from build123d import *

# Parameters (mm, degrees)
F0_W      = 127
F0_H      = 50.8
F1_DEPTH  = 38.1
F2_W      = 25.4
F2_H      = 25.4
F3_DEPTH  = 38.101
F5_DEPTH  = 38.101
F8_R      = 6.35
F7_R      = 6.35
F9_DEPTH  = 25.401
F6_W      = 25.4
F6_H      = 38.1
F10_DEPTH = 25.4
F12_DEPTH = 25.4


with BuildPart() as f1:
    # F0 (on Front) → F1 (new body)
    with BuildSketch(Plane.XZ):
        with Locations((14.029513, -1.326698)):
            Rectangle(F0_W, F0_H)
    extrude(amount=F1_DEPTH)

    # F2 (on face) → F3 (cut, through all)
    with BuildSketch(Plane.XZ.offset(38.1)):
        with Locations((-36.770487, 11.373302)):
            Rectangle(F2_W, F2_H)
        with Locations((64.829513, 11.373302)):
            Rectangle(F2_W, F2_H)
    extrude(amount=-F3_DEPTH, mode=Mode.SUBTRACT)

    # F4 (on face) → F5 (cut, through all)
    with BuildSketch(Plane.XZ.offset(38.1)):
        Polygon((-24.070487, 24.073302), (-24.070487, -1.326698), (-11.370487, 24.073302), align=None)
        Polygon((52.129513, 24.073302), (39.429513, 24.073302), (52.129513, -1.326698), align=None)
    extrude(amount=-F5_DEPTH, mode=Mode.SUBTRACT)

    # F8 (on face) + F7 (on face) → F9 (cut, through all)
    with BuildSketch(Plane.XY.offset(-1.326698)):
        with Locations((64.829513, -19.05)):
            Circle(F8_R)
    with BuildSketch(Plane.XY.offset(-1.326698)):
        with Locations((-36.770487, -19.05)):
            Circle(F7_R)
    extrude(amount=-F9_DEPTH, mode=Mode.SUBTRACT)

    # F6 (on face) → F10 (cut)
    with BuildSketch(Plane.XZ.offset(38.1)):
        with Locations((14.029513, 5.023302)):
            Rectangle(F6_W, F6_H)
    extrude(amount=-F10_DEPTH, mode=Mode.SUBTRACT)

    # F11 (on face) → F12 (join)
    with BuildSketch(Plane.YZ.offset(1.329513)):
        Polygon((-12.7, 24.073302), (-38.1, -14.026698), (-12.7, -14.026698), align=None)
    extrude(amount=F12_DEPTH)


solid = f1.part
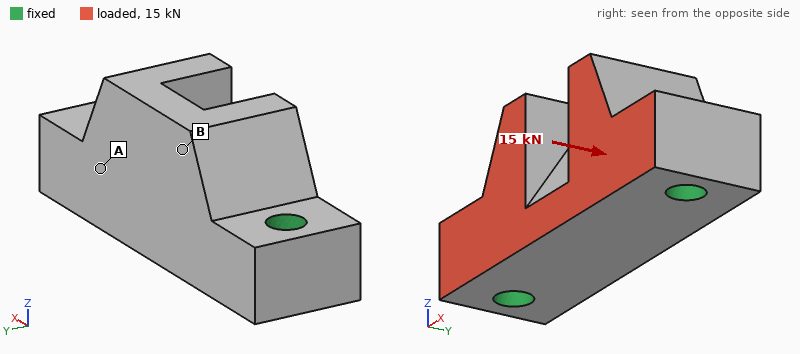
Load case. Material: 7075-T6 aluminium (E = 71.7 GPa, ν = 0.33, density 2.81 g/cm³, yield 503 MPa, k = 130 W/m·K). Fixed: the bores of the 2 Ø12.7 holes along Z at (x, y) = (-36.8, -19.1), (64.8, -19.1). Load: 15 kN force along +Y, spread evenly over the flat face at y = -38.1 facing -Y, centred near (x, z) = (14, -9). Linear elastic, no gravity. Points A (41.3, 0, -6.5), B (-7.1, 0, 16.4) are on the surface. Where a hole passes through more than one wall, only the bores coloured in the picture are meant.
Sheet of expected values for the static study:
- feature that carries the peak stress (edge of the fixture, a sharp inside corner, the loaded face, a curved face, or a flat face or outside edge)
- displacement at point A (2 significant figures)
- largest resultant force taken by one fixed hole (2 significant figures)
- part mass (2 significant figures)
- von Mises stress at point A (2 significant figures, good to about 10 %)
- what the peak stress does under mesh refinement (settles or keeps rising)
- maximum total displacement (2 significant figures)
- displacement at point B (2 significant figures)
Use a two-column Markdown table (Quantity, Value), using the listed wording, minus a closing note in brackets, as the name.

| Quantity | Value |
|---|---|
| feature that carries the peak stress | edge of the fixture |
| displacement at point A | 11 µm |
| largest resultant force taken by one fixed hole | 7.5 kN |
| part mass | 470 g |
| von Mises stress at point A | 8.8 MPa |
| what the peak stress does under mesh refinement | keeps rising |
| maximum total displacement | 23 µm |
| displacement at point B | 18 µm |
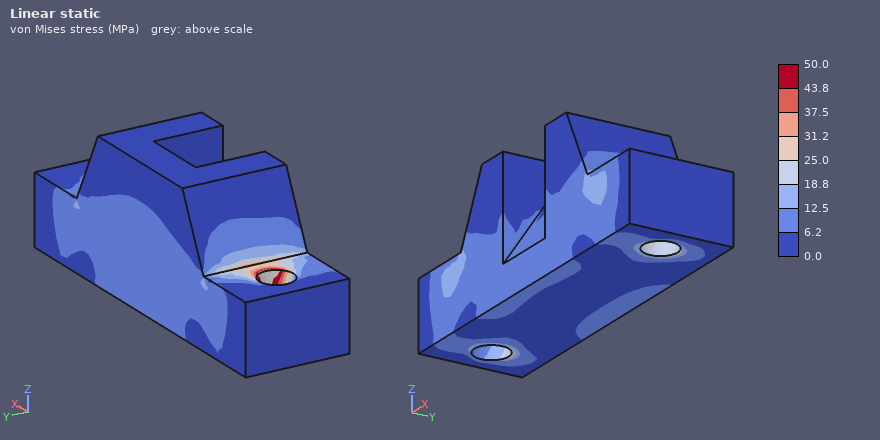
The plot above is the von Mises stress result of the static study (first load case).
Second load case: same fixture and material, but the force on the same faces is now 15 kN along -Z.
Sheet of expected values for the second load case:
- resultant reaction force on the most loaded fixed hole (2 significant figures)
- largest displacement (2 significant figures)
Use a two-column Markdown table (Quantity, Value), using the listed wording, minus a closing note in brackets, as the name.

| Quantity | Value |
|---|---|
| resultant reaction force on the most loaded fixed hole | 7.6 kN |
| largest displacement | 35 µm |
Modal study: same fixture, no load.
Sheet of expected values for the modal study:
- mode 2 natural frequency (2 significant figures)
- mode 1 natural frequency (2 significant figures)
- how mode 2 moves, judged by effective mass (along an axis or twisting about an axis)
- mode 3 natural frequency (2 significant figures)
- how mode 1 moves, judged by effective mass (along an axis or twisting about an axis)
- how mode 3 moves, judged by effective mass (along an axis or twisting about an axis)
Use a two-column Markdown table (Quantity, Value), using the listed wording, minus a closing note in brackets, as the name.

| Quantity | Value |
|---|---|
| mode 2 natural frequency | 9600 Hz |
| mode 1 natural frequency | 6500 Hz |
| how mode 2 moves, judged by effective mass | along Z |
| mode 3 natural frequency | 11 kHz |
| how mode 1 moves, judged by effective mass | along Y |
| how mode 3 moves, judged by effective mass | along Y |
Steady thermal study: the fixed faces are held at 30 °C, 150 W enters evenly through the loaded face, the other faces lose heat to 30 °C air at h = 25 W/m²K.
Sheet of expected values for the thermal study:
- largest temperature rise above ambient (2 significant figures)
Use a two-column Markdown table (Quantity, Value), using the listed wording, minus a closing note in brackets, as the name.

| Quantity | Value |
|---|---|
| largest temperature rise above ambient | 15 K |
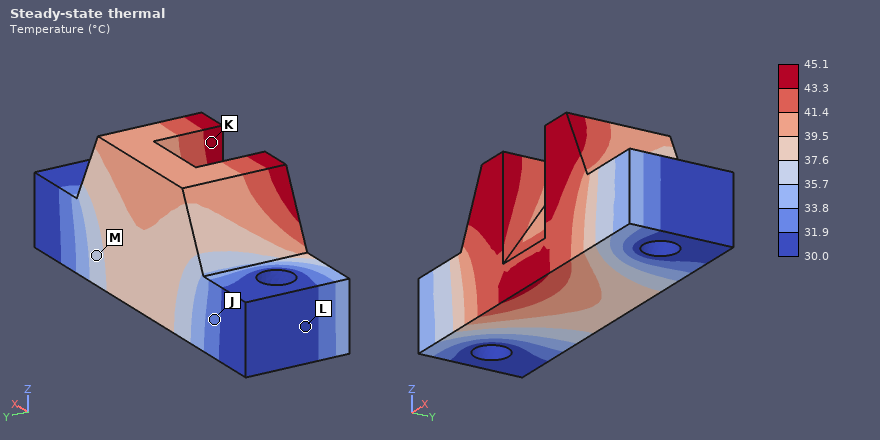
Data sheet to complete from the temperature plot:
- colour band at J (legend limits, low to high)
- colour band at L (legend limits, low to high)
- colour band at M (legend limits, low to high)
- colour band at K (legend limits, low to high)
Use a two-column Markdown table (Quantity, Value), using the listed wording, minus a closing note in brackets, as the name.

| Quantity | Value |
|---|---|
| colour band at J | 31.9 to 33.8 °C |
| colour band at L | 30.0 to 31.9 °C |
| colour band at M | 35.7 to 37.6 °C |
| colour band at K | 43.3 to 45.1 °C |
